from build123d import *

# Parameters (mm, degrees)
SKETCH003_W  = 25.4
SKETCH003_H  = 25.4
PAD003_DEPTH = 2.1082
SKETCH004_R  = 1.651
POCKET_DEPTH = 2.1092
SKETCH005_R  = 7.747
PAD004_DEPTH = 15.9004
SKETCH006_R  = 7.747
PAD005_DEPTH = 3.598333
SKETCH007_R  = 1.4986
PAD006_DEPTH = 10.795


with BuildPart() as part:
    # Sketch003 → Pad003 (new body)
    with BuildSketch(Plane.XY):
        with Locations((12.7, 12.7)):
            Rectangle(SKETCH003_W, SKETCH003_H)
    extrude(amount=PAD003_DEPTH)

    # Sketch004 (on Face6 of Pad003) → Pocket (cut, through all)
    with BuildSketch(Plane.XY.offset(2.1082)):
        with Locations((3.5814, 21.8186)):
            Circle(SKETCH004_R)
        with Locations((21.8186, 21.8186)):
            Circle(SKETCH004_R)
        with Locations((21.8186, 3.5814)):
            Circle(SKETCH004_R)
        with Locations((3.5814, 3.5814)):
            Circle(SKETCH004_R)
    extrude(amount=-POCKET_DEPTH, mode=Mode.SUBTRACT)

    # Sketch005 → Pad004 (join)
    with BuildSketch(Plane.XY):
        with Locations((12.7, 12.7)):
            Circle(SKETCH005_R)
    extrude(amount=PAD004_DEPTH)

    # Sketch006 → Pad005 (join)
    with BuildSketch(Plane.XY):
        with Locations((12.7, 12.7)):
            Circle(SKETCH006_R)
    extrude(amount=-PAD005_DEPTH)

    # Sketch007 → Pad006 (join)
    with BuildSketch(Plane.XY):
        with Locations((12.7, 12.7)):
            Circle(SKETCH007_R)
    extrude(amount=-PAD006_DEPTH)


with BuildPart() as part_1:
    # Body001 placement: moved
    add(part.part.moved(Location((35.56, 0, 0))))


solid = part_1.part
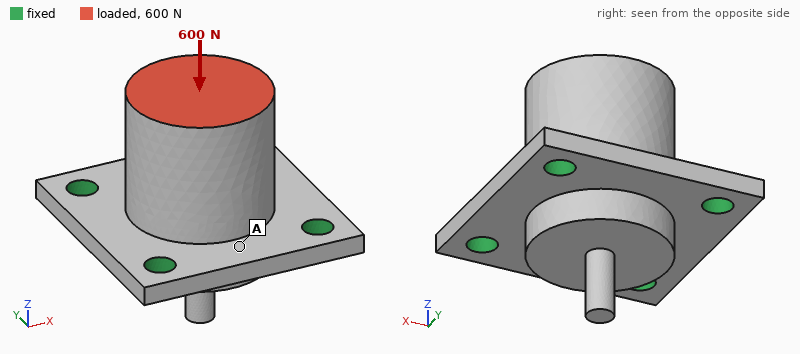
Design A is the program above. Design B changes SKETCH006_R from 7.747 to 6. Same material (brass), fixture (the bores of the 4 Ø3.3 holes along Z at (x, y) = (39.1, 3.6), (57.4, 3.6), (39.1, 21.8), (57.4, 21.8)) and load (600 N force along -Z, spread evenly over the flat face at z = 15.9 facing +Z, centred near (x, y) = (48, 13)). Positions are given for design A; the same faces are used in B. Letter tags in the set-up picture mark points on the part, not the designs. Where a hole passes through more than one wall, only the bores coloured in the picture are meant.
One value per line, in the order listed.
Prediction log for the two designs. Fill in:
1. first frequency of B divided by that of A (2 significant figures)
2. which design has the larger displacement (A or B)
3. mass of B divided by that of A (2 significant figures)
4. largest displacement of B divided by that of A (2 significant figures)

0.96
B
0.94
1.1
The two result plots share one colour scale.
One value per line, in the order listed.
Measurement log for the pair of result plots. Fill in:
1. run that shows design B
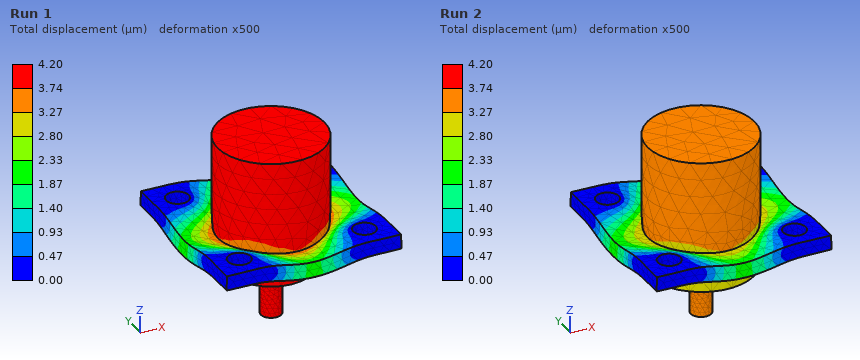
Run 1
